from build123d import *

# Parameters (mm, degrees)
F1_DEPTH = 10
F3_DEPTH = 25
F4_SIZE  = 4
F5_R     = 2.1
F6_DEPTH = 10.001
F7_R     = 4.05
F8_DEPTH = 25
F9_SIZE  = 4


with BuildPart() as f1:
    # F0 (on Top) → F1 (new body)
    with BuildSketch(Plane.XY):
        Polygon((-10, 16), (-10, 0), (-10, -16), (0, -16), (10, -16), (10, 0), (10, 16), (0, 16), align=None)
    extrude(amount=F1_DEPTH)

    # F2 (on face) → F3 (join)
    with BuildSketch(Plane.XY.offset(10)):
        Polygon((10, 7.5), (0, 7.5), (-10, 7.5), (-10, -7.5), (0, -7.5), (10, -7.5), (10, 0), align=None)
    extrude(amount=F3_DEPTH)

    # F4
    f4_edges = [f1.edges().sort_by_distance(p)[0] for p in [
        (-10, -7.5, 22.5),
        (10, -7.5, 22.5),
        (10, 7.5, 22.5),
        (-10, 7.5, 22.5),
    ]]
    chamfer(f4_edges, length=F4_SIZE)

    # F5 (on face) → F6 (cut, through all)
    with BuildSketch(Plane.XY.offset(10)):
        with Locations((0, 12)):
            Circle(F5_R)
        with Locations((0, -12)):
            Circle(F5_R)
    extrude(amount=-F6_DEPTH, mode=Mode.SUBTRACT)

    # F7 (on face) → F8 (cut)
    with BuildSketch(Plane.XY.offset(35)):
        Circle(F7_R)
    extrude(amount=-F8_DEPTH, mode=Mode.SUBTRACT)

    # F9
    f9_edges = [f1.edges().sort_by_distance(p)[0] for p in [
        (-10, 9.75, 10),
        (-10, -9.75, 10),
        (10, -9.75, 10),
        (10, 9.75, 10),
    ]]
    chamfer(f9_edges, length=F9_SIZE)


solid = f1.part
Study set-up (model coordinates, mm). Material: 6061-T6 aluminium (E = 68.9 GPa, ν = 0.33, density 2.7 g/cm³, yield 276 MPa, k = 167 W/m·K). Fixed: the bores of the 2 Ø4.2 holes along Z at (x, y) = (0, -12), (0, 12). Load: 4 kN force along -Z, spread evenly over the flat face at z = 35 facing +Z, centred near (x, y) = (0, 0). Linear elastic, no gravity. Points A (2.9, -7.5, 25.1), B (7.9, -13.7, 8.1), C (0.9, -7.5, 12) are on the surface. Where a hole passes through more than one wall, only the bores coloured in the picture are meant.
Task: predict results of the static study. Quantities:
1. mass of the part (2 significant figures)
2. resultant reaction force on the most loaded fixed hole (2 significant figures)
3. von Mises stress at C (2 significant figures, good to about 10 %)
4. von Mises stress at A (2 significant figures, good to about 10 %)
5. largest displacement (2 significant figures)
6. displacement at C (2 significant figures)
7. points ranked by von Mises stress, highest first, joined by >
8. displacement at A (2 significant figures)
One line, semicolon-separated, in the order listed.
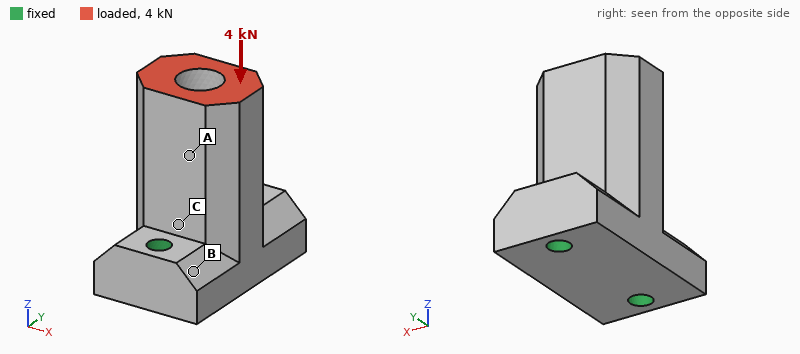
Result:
30 g; 2.0 kN; 33 MPa; 19 MPa; 12 µm; 5.2 µm; C > A > B; 9.3 µm
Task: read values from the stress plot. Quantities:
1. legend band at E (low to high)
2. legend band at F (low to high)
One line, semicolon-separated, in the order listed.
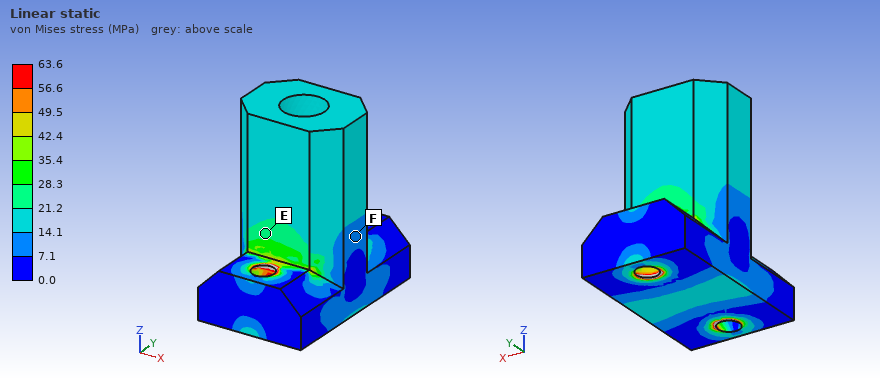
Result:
21.2 to 28.3 MPa; 7.1 to 14.1 MPa
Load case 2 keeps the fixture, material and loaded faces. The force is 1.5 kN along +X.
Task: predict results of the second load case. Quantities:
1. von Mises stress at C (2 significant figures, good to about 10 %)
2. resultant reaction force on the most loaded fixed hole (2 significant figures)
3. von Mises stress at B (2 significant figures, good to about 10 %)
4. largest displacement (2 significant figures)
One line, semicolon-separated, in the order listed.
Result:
37 MPa; 750 N; 18 MPa; 90 µm
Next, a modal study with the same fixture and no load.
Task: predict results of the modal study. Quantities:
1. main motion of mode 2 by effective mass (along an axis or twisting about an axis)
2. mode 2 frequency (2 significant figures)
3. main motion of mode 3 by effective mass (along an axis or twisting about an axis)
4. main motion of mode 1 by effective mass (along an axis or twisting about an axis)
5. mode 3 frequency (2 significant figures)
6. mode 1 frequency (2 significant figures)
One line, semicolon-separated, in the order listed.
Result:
along Y; 12 kHz; twisting about Z; along X; 26 kHz; 8700 Hz
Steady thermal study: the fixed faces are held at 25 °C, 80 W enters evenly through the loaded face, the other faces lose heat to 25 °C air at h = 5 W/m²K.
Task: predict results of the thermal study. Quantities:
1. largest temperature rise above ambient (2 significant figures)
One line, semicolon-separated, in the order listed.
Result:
70 K
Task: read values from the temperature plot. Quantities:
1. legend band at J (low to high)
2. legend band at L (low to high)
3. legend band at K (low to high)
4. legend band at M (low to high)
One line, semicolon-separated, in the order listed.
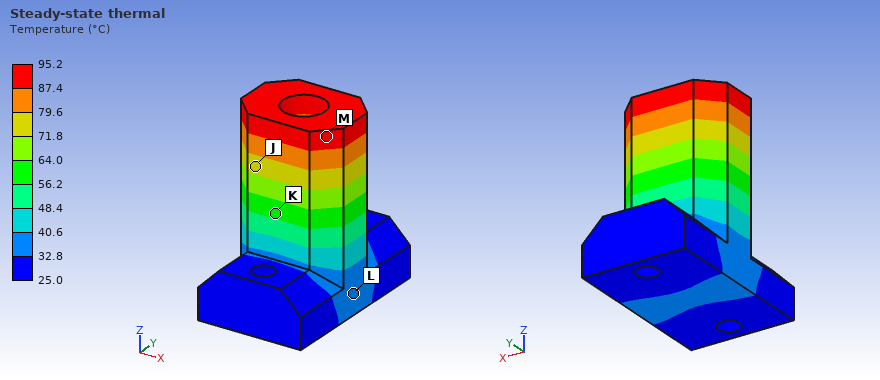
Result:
71.8 to 79.6 °C; 32.8 to 40.6 °C; 56.2 to 64.0 °C; 87.4 to 95.2 °C
